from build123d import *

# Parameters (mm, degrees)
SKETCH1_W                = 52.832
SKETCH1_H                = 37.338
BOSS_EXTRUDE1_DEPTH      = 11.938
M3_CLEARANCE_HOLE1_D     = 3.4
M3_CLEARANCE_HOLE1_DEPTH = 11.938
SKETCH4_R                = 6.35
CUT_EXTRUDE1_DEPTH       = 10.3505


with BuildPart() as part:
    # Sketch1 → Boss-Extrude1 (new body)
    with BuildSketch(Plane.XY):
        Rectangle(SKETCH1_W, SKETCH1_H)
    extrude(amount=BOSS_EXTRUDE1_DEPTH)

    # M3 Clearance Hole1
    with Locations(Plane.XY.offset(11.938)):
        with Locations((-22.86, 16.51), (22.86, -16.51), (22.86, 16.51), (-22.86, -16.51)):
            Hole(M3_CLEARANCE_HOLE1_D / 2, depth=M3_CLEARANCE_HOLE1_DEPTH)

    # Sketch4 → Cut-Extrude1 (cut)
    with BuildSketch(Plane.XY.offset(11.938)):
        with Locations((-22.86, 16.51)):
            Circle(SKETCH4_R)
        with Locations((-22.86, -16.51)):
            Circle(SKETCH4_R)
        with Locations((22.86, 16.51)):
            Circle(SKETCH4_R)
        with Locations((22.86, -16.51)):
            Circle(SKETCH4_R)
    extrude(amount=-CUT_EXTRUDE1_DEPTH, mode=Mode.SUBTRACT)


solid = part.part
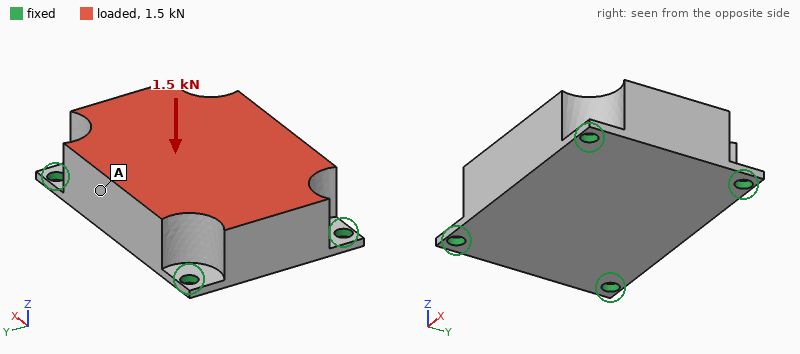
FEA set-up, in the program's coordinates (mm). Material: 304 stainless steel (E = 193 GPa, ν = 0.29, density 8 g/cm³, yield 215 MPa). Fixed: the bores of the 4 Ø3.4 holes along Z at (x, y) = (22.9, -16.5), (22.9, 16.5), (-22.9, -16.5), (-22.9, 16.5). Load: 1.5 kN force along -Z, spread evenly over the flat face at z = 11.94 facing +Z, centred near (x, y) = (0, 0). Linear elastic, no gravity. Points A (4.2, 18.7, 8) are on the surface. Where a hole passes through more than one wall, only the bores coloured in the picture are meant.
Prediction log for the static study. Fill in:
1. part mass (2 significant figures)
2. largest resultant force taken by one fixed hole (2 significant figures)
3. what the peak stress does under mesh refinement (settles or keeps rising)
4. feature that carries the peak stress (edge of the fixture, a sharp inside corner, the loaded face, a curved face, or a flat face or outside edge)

160 g
430 N
keeps rising
edge of the fixture
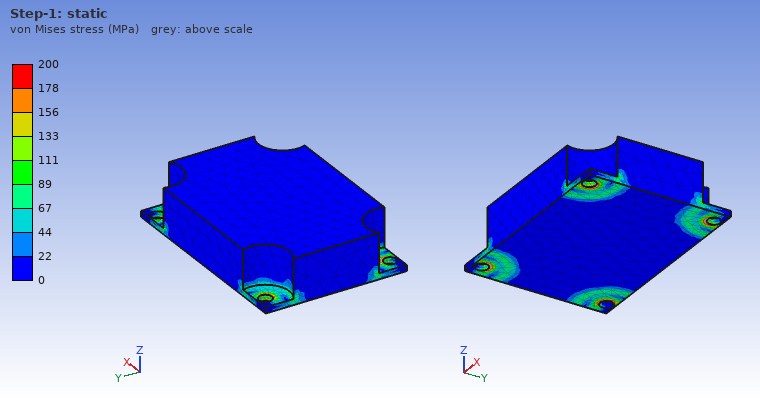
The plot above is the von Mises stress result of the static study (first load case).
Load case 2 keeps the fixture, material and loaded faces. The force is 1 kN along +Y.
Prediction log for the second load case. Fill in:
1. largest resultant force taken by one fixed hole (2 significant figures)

330 N
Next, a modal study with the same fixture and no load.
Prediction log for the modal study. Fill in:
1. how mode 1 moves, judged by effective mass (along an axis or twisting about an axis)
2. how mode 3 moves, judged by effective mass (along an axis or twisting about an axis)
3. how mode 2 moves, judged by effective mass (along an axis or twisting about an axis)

along Z
along X
along Y
